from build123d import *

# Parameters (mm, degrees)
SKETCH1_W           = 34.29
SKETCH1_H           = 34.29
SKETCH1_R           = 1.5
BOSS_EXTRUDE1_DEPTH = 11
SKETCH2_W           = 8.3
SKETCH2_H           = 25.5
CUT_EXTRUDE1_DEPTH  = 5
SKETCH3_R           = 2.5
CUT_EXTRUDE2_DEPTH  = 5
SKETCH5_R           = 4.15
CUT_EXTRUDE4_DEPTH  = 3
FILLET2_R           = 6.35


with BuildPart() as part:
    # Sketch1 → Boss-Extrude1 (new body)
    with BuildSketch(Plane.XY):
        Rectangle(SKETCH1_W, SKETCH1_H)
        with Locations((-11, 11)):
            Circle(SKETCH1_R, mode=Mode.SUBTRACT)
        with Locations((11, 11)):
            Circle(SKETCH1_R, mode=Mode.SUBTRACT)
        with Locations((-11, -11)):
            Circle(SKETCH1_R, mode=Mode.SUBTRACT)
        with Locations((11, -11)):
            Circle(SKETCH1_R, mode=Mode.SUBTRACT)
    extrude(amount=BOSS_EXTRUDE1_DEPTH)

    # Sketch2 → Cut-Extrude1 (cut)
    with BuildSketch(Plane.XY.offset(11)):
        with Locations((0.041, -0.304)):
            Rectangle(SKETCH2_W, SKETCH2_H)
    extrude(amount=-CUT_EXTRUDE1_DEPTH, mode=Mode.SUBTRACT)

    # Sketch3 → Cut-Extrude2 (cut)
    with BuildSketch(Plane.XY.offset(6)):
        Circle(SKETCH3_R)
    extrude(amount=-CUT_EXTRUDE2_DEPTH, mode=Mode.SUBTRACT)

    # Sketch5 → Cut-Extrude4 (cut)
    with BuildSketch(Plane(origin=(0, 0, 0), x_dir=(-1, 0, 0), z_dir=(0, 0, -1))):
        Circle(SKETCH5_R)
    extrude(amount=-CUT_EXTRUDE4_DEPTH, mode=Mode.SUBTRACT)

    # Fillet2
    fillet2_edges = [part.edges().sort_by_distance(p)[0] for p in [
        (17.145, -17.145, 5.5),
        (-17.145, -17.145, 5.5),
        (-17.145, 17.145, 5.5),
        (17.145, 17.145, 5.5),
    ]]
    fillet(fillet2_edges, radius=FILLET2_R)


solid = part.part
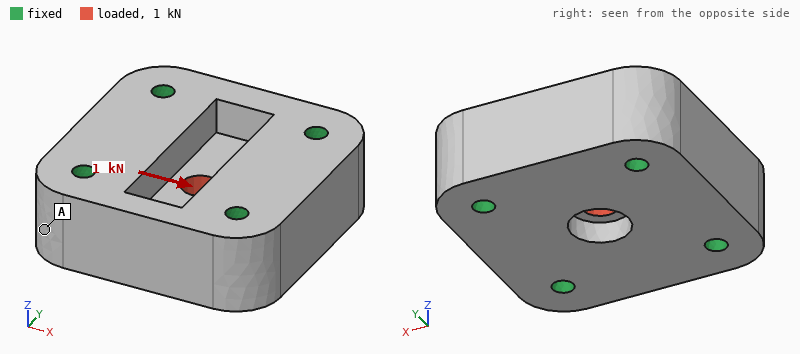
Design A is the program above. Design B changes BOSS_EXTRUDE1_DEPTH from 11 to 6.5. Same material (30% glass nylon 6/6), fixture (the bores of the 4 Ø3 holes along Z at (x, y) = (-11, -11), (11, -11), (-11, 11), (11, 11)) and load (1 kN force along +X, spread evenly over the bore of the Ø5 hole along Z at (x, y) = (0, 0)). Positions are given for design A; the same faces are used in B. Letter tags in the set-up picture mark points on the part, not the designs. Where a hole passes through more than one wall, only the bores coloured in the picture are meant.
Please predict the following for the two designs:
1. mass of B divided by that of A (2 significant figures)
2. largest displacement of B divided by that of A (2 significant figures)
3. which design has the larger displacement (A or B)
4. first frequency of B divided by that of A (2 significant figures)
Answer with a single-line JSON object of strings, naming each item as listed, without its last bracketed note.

{"mass of B divided by that of A": "0.63", "largest displacement of B divided by that of A": "1.2", "which design has the larger displacement": "B", "first frequency of B divided by that of A": "0.80"}
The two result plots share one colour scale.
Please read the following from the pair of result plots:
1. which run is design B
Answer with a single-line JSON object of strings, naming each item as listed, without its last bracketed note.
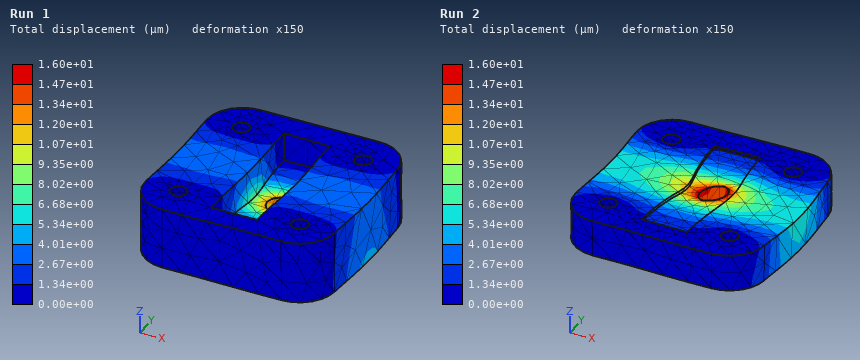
{"which run is design B": "Run 2"}
